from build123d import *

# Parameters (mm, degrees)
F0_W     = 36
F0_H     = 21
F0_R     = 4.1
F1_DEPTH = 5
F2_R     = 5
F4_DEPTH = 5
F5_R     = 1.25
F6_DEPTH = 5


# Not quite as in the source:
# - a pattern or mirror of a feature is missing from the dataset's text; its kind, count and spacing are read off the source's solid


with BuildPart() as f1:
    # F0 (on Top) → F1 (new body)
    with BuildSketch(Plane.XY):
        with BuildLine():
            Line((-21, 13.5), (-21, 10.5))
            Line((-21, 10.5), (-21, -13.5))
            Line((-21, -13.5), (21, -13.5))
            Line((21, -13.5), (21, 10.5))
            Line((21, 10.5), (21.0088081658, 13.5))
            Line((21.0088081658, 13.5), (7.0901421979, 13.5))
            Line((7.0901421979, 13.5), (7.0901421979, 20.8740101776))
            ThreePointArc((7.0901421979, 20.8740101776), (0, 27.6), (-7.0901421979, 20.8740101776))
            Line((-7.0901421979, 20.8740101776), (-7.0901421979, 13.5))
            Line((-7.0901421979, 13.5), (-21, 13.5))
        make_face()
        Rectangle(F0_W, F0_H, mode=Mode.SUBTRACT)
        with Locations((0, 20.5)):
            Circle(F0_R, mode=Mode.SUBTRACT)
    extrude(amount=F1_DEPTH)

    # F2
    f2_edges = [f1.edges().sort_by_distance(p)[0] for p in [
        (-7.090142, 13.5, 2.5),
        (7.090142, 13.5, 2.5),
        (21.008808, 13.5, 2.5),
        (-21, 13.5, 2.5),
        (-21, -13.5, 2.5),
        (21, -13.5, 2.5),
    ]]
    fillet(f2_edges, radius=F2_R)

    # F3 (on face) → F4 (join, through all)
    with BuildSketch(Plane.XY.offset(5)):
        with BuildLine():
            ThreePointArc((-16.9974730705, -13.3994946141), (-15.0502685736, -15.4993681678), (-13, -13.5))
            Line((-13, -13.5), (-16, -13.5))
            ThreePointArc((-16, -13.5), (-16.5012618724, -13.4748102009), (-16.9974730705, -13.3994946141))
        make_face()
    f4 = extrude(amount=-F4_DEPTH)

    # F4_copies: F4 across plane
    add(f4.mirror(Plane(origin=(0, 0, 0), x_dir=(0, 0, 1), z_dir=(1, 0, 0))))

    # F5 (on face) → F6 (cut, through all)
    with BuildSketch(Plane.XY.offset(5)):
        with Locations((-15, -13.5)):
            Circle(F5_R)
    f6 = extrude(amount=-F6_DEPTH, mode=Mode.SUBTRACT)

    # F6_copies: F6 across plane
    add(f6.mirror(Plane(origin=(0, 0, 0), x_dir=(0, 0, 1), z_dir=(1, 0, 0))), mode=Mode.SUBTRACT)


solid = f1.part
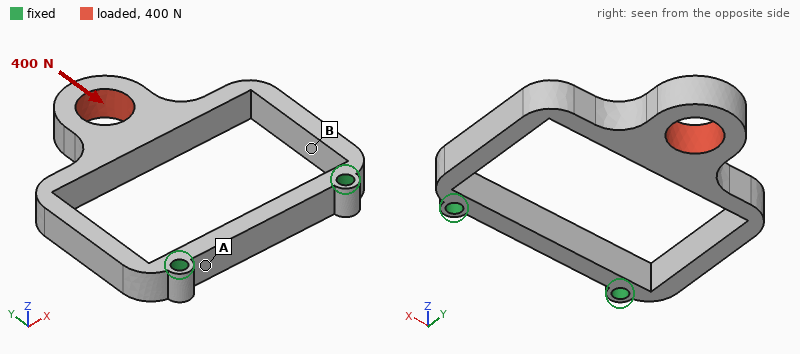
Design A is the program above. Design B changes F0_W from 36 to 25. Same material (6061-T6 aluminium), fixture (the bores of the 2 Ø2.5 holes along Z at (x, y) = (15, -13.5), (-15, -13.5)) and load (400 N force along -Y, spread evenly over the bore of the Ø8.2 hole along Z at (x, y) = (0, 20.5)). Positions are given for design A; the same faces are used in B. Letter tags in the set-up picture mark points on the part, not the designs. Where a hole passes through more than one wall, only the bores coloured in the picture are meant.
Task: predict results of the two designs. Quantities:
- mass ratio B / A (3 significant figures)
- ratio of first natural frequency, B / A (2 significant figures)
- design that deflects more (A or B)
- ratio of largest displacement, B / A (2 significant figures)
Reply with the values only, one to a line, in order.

1.47
1.9
A
0.17
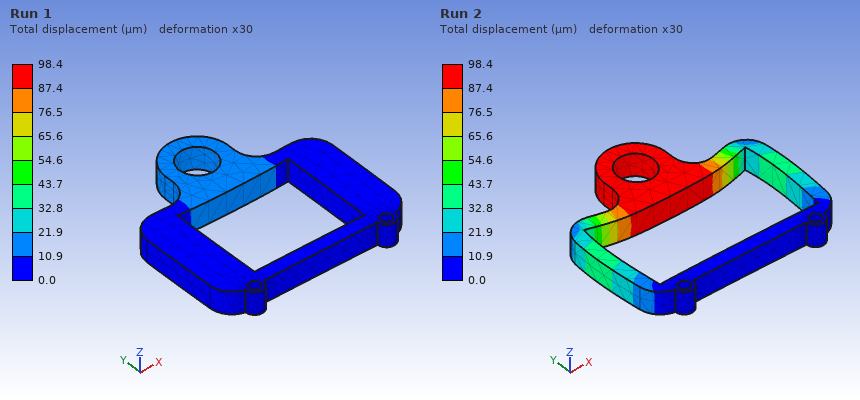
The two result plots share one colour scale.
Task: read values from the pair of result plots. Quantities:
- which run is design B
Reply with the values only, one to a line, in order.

Run 1
